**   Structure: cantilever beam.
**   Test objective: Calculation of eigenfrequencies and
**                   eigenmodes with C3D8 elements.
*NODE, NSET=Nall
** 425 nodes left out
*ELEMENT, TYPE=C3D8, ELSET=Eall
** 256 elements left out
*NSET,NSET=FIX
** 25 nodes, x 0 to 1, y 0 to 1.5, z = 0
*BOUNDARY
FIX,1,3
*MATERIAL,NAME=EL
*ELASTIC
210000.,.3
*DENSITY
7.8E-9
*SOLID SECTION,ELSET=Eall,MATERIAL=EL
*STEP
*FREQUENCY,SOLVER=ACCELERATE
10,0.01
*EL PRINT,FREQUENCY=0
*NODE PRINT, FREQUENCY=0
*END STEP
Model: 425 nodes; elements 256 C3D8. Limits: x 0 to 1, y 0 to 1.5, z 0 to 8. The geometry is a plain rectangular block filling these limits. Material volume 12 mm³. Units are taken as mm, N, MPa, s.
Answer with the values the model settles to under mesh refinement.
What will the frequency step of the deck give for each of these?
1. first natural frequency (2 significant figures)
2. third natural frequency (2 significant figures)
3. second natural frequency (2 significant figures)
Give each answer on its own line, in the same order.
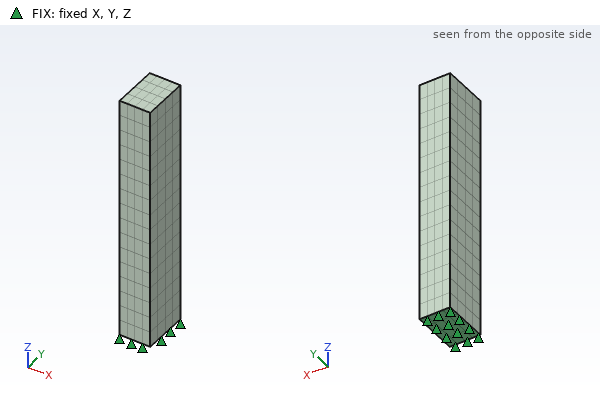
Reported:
13000 Hz
76000 Hz
19000 Hz
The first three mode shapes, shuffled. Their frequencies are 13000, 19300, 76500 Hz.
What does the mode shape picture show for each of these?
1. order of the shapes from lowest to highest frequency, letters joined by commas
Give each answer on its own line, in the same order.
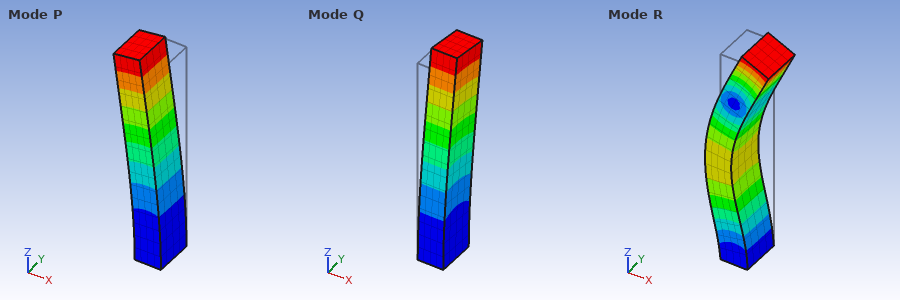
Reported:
P, Q, R
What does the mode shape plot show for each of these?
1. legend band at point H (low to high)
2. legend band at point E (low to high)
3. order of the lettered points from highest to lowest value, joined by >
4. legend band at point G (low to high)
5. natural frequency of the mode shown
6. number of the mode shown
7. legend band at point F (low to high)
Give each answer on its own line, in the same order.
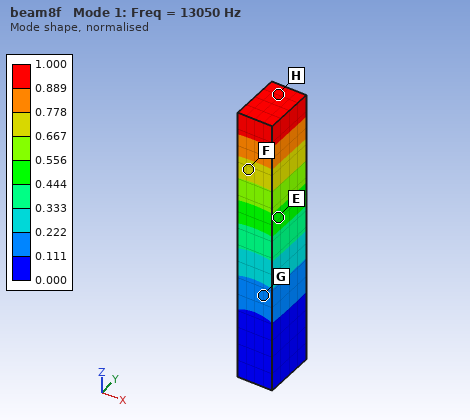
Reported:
0.889 to 1.000
0.444 to 0.556
H > F > E > G
0.111 to 0.222
13050 Hz
1
0.667 to 0.778
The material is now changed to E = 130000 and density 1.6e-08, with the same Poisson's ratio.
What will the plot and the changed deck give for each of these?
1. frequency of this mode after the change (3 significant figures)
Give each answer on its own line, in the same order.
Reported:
7170 Hz
